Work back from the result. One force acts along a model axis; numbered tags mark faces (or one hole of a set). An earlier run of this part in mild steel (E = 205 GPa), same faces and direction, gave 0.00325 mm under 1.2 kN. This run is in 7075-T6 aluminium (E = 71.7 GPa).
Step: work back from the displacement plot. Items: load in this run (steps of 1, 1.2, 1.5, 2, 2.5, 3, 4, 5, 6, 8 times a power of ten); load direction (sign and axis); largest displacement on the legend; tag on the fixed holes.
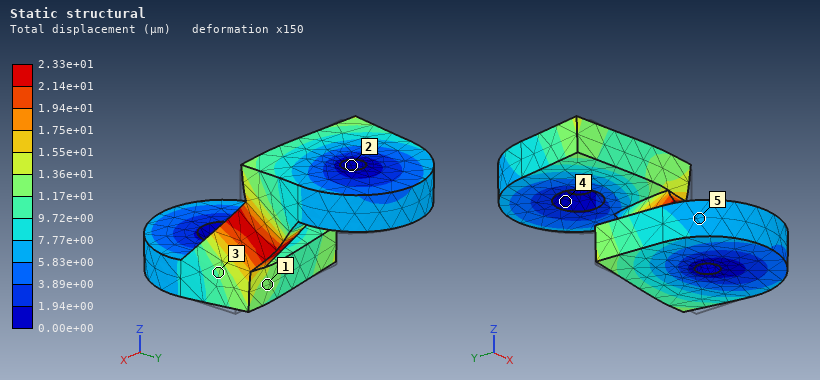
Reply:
3 kN
-X
2.33e+01 µm
2
